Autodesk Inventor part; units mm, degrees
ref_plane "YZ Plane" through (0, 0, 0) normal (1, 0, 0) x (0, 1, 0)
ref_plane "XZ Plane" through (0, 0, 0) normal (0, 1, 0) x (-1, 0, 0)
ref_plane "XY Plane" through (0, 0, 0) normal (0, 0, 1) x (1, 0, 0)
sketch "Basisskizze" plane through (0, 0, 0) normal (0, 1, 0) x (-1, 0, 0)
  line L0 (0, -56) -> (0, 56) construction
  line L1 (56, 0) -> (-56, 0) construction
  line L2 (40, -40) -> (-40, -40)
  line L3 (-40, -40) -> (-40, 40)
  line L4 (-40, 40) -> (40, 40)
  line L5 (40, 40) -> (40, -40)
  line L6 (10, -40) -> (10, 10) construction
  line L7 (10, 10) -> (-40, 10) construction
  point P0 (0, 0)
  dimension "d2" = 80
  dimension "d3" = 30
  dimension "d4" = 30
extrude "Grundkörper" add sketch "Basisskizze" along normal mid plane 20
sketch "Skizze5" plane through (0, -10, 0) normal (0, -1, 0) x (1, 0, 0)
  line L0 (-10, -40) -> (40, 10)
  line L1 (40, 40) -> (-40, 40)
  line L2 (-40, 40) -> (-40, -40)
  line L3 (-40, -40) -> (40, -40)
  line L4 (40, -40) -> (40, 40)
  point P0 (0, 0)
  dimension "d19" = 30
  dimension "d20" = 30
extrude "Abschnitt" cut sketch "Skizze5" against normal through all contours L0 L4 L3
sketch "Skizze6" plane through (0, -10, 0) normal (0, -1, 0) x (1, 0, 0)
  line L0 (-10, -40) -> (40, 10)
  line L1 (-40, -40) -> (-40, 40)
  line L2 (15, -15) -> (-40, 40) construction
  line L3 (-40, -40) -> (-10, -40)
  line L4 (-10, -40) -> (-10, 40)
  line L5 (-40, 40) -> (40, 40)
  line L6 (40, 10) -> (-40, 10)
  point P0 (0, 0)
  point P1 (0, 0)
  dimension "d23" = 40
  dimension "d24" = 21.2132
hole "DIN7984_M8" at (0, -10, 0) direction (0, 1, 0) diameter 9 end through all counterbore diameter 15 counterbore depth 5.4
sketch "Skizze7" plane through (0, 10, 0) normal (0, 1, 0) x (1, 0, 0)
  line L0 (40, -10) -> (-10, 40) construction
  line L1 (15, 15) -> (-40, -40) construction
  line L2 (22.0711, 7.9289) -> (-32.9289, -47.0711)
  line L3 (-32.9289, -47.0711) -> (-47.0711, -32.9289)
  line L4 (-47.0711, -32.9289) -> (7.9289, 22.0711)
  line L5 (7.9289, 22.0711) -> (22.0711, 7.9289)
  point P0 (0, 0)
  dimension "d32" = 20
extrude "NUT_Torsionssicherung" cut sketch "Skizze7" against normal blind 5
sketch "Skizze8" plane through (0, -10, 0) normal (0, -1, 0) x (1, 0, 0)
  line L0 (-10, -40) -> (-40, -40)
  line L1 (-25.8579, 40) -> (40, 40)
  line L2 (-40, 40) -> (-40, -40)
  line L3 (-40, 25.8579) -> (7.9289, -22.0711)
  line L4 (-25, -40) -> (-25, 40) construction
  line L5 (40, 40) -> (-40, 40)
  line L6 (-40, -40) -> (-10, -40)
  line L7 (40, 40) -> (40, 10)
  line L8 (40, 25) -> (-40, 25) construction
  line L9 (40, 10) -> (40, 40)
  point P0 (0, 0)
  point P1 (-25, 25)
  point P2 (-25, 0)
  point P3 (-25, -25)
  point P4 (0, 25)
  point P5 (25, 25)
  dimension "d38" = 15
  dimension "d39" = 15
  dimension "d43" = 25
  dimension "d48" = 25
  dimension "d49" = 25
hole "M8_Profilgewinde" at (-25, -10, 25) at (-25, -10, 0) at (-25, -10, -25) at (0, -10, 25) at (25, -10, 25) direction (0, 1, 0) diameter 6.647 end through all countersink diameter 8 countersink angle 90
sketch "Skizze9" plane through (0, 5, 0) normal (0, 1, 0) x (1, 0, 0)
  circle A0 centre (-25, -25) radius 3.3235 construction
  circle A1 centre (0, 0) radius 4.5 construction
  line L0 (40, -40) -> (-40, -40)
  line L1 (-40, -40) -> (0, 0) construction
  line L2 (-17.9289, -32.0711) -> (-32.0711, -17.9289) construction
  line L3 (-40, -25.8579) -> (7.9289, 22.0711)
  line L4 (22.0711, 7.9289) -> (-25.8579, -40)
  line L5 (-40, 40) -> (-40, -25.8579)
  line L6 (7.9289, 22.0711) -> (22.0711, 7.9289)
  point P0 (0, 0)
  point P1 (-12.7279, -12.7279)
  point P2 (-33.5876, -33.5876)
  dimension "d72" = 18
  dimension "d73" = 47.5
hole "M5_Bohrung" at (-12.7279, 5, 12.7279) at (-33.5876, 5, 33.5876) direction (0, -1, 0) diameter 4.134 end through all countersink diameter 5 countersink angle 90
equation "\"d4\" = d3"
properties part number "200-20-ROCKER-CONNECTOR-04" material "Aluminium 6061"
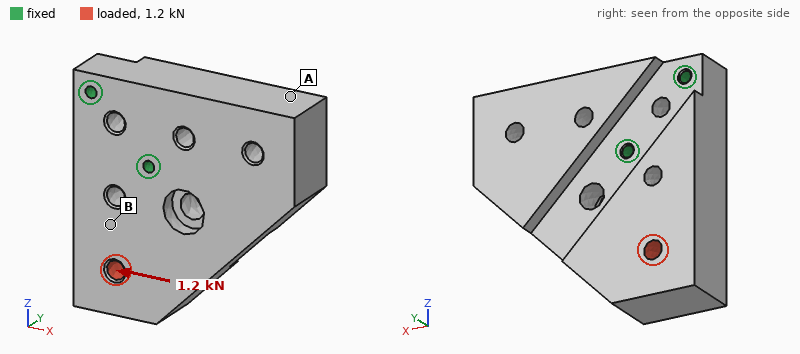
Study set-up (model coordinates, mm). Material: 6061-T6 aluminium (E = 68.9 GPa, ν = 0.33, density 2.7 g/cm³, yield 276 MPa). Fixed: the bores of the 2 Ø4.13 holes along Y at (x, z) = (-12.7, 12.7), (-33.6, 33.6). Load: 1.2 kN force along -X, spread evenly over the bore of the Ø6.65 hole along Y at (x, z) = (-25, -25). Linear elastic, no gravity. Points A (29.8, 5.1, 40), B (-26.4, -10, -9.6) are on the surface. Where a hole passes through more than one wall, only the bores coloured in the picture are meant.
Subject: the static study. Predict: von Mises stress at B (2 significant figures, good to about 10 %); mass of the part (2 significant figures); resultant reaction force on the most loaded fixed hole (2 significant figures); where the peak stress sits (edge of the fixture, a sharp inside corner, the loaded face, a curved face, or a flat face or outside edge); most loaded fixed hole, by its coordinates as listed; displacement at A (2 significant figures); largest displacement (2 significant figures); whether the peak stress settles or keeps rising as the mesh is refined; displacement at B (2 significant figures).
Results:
3.9 MPa
240 g
2.3 kN
edge of the fixture
(-12.7, 12.7)
8.3 µm
14 µm
keeps rising
5.7 µm
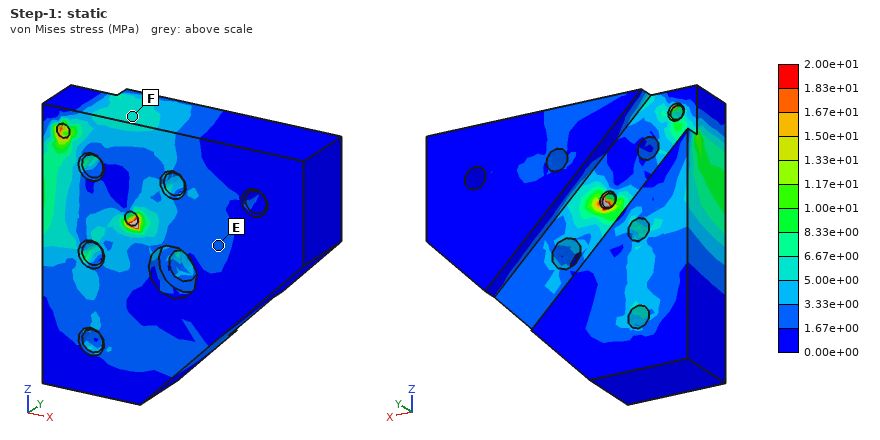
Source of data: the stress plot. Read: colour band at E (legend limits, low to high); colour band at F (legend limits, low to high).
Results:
1.67e+00 to 3.33e+00 MPa
5.00e+00 to 6.67e+00 MPa
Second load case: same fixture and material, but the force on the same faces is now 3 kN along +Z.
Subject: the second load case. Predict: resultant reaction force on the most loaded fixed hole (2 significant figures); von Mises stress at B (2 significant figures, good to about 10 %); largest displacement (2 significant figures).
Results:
1.6 kN
4.1 MPa
12 µm
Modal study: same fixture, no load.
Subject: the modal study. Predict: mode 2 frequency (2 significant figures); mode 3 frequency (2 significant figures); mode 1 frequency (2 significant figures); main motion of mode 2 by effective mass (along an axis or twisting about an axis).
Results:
3700 Hz
4800 Hz
2900 Hz
along Y
